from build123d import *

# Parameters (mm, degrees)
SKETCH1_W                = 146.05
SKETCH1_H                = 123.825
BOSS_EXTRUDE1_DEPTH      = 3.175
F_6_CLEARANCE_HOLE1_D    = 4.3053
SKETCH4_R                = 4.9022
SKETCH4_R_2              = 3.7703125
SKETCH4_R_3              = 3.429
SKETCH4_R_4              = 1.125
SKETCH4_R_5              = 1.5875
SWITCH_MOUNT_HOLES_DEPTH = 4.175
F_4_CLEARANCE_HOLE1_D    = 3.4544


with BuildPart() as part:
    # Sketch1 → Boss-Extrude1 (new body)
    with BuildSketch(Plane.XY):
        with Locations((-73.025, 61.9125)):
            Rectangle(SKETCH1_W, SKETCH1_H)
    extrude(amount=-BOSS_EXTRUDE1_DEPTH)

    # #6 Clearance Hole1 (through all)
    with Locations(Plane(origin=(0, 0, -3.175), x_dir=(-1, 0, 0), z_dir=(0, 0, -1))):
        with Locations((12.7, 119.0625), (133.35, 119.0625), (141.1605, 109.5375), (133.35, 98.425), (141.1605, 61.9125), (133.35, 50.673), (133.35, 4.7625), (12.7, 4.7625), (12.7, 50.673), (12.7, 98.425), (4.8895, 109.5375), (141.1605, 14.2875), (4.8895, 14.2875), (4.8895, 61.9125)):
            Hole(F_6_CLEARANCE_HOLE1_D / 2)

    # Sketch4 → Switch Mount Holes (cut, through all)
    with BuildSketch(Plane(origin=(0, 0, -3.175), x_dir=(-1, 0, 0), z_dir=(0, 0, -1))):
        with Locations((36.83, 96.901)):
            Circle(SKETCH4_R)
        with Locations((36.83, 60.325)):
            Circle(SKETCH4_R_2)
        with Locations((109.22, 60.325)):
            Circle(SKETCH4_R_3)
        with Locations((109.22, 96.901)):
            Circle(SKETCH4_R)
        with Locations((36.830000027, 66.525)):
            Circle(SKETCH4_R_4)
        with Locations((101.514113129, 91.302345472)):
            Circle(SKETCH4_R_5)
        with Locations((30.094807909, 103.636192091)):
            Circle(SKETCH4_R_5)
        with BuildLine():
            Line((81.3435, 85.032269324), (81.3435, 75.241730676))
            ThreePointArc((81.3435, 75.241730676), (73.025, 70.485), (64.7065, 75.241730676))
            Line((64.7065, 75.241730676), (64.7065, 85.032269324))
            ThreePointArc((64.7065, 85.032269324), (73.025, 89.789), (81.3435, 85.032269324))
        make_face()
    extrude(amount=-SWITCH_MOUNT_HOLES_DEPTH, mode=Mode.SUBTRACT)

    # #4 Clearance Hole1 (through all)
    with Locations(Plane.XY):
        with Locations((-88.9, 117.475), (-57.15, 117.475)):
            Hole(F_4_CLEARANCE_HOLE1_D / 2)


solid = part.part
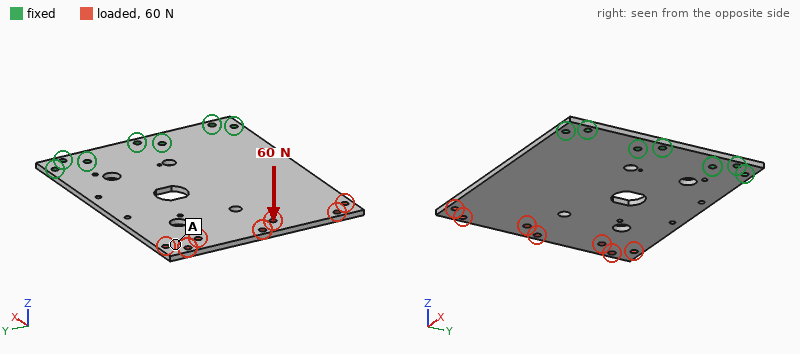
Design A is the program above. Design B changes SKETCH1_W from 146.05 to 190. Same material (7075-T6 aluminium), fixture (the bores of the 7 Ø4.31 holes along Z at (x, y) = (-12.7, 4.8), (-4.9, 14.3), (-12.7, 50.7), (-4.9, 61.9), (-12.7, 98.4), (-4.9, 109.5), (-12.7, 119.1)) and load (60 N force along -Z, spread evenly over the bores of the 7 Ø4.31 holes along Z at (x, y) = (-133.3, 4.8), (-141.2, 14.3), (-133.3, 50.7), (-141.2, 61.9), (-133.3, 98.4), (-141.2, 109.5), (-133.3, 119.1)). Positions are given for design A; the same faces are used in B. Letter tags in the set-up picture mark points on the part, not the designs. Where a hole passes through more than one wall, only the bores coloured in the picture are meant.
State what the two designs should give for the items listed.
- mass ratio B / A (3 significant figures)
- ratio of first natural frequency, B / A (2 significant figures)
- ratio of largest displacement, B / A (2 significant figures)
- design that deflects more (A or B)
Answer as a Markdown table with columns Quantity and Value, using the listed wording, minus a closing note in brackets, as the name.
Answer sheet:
| Quantity | Value |
|---|---|
| mass ratio B / A | 1.31 |
| ratio of first natural frequency, B / A | 0.73 |
| ratio of largest displacement, B / A | 1.2 |
| design that deflects more | B |
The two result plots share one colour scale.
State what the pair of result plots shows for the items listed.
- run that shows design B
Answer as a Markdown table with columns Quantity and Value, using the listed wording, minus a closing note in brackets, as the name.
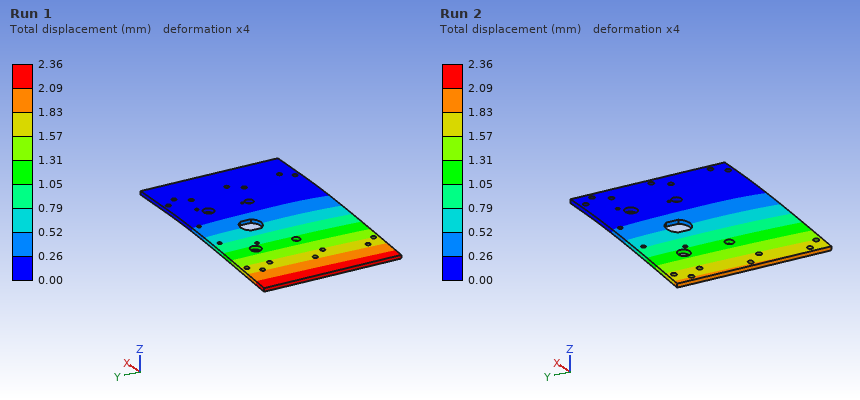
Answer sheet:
| Quantity | Value |
|---|---|
| run that shows design B | Run 1 |
